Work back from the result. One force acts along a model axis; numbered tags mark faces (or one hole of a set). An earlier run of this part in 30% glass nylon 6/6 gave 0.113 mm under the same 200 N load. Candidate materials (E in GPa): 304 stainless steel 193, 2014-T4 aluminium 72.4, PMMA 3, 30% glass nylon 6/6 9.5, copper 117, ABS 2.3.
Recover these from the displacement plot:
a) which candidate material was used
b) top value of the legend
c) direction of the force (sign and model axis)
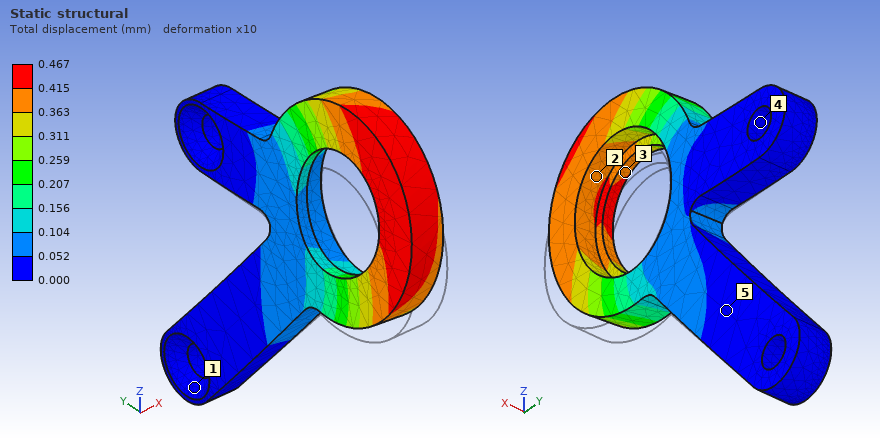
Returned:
ABS
0.467 mm
+Z
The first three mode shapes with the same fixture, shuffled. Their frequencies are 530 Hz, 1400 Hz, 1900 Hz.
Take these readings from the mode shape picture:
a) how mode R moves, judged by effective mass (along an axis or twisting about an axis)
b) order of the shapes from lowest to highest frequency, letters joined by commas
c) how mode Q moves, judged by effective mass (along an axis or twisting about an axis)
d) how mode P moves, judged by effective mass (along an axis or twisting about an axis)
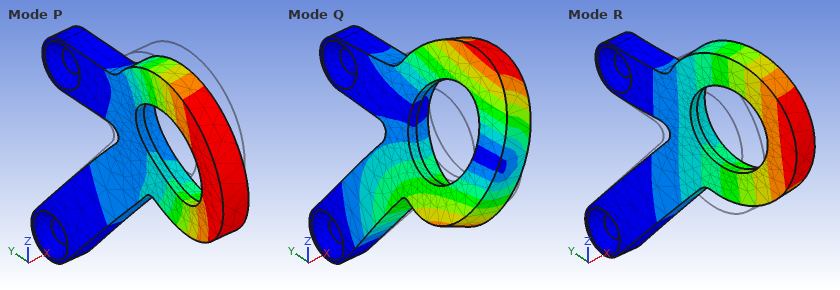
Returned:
along X
R, Q, P
twisting about Y
along Z
